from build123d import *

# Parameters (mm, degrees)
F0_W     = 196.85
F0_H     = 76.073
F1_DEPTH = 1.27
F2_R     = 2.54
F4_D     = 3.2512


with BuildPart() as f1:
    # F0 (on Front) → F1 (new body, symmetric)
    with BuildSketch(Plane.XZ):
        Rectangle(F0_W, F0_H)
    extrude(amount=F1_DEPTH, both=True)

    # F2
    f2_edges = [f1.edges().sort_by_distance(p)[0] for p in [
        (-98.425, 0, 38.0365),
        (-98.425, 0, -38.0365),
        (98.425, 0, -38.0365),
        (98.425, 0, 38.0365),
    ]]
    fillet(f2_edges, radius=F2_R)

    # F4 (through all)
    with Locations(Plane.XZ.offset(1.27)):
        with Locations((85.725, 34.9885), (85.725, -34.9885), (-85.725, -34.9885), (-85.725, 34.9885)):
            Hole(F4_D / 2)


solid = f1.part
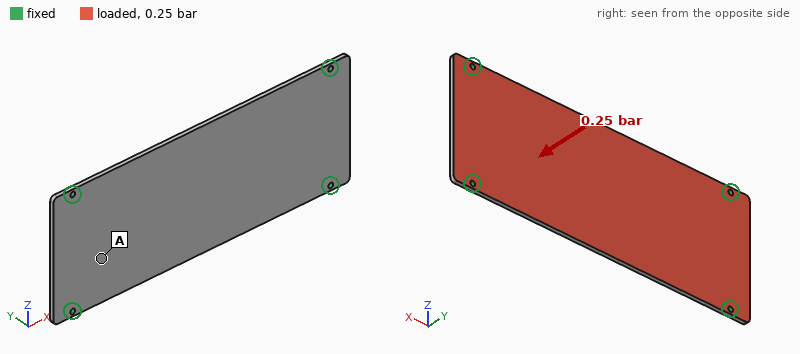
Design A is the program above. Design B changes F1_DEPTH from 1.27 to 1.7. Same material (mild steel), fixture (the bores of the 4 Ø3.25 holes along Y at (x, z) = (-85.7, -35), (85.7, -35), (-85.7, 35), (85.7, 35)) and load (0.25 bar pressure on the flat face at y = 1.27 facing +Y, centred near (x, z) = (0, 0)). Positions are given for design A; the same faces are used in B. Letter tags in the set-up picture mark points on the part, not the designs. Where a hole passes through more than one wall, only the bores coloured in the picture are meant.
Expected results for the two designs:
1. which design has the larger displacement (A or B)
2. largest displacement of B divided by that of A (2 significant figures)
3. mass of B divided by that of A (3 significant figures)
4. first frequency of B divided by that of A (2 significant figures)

A
0.43
1.34
1.3
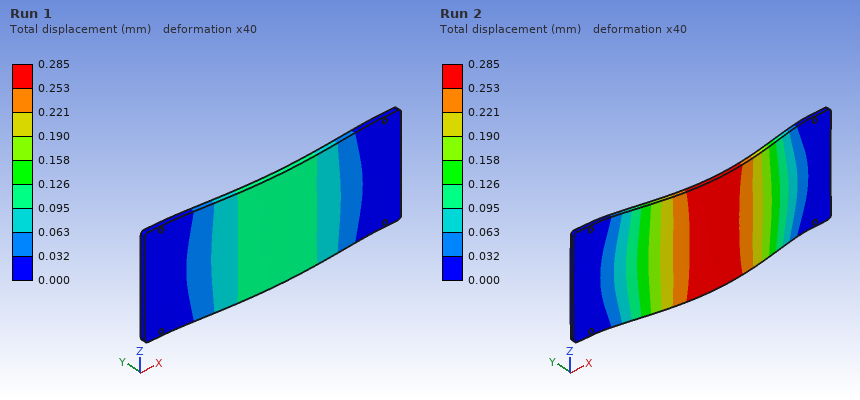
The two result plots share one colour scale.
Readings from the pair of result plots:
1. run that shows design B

Run 1
